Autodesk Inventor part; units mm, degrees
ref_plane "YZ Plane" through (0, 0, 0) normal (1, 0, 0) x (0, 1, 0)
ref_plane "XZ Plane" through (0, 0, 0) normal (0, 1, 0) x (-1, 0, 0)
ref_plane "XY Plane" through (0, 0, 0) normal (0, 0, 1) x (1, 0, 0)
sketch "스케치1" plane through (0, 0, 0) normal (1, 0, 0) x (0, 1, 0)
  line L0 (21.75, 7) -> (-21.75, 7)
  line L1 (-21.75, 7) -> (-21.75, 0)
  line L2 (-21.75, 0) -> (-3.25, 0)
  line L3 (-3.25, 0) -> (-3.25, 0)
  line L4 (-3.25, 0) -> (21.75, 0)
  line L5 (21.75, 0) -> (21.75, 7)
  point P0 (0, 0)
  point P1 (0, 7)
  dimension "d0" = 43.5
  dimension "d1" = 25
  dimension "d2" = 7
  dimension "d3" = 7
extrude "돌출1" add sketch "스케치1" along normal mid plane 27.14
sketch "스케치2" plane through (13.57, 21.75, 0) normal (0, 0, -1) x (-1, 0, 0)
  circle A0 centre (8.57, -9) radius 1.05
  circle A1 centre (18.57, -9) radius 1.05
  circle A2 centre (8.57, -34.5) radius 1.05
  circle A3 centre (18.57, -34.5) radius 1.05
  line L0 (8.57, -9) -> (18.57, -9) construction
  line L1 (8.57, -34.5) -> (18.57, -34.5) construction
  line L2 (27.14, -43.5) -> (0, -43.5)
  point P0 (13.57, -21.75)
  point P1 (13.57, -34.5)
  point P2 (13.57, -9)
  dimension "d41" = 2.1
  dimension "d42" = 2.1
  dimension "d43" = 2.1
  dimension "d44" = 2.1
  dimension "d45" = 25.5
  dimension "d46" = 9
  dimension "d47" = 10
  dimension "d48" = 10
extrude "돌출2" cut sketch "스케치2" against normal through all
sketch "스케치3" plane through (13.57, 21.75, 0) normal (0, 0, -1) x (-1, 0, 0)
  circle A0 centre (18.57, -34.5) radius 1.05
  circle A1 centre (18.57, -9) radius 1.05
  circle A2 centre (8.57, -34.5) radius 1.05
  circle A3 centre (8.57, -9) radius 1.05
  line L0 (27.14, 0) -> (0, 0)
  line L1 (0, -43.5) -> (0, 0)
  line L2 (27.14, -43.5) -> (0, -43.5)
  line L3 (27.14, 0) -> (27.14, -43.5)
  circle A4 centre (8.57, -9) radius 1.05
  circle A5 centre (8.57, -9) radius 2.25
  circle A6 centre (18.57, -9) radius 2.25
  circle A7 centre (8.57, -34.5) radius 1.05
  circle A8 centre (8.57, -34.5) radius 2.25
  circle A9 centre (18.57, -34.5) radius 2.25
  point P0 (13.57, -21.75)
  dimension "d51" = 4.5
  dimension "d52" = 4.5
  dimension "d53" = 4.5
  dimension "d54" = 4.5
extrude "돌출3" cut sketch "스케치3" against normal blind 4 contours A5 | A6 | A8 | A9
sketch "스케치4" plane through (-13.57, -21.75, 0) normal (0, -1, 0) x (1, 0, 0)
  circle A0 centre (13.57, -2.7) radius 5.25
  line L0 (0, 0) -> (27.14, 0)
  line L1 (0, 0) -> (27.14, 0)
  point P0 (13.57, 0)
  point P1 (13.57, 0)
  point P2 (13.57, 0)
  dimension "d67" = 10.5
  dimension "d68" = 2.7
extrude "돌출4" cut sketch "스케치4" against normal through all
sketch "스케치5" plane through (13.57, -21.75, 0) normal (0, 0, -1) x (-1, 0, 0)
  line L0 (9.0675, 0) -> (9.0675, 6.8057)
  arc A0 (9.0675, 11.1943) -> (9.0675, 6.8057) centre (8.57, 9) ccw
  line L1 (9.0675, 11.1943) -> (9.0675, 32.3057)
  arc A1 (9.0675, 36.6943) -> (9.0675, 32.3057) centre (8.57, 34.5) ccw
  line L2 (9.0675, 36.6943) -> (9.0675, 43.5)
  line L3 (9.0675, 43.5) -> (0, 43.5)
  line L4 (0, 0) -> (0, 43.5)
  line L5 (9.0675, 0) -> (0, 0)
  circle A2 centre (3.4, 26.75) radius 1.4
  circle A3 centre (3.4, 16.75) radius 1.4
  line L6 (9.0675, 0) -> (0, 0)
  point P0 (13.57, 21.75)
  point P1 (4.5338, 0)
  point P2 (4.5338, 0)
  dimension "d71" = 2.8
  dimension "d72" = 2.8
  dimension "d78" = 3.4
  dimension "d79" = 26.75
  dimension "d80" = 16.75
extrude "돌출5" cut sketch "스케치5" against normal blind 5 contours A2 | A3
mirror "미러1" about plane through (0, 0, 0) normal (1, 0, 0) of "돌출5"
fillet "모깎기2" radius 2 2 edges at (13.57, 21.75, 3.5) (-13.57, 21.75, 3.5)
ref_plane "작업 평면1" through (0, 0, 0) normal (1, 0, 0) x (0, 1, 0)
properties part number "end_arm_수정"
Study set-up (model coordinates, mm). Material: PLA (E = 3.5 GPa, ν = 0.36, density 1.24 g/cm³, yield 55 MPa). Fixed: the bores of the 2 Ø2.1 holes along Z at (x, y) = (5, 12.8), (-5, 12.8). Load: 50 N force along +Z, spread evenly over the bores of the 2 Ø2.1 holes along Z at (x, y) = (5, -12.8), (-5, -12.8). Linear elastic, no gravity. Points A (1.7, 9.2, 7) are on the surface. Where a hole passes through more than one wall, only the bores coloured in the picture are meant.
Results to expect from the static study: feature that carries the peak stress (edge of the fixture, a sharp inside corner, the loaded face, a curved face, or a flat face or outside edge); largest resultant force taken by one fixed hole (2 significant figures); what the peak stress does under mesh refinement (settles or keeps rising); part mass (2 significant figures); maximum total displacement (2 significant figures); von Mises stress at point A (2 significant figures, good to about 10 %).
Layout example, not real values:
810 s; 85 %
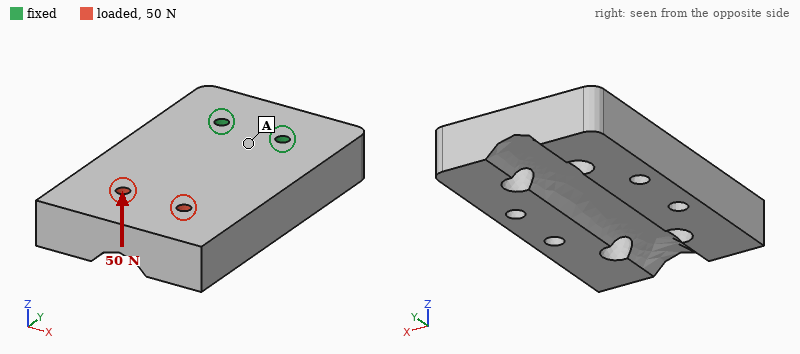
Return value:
edge of the fixture; 25 N; keeps rising; 8.9 g; 0.60 mm; 7.3 MPa
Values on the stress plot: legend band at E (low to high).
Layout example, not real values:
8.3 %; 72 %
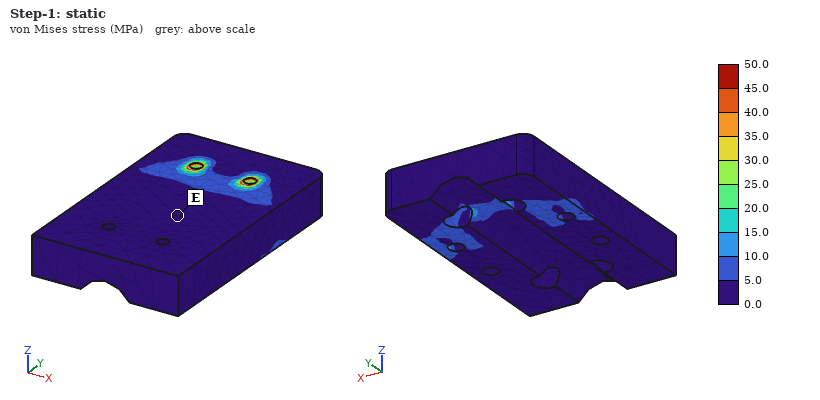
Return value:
0.0 to 5.0 MPa
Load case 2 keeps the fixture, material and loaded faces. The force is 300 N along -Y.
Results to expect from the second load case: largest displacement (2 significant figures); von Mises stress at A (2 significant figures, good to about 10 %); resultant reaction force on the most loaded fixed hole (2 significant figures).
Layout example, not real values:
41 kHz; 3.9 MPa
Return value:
0.12 mm; 4.1 MPa; 150 N
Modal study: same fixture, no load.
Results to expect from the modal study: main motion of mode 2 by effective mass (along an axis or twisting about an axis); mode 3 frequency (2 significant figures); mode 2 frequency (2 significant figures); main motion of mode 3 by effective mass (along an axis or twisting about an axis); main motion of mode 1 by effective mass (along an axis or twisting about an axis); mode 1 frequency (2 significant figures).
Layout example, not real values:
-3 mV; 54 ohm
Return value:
along X; 2700 Hz; 2500 Hz; twisting about Y; along Z; 830 Hz
